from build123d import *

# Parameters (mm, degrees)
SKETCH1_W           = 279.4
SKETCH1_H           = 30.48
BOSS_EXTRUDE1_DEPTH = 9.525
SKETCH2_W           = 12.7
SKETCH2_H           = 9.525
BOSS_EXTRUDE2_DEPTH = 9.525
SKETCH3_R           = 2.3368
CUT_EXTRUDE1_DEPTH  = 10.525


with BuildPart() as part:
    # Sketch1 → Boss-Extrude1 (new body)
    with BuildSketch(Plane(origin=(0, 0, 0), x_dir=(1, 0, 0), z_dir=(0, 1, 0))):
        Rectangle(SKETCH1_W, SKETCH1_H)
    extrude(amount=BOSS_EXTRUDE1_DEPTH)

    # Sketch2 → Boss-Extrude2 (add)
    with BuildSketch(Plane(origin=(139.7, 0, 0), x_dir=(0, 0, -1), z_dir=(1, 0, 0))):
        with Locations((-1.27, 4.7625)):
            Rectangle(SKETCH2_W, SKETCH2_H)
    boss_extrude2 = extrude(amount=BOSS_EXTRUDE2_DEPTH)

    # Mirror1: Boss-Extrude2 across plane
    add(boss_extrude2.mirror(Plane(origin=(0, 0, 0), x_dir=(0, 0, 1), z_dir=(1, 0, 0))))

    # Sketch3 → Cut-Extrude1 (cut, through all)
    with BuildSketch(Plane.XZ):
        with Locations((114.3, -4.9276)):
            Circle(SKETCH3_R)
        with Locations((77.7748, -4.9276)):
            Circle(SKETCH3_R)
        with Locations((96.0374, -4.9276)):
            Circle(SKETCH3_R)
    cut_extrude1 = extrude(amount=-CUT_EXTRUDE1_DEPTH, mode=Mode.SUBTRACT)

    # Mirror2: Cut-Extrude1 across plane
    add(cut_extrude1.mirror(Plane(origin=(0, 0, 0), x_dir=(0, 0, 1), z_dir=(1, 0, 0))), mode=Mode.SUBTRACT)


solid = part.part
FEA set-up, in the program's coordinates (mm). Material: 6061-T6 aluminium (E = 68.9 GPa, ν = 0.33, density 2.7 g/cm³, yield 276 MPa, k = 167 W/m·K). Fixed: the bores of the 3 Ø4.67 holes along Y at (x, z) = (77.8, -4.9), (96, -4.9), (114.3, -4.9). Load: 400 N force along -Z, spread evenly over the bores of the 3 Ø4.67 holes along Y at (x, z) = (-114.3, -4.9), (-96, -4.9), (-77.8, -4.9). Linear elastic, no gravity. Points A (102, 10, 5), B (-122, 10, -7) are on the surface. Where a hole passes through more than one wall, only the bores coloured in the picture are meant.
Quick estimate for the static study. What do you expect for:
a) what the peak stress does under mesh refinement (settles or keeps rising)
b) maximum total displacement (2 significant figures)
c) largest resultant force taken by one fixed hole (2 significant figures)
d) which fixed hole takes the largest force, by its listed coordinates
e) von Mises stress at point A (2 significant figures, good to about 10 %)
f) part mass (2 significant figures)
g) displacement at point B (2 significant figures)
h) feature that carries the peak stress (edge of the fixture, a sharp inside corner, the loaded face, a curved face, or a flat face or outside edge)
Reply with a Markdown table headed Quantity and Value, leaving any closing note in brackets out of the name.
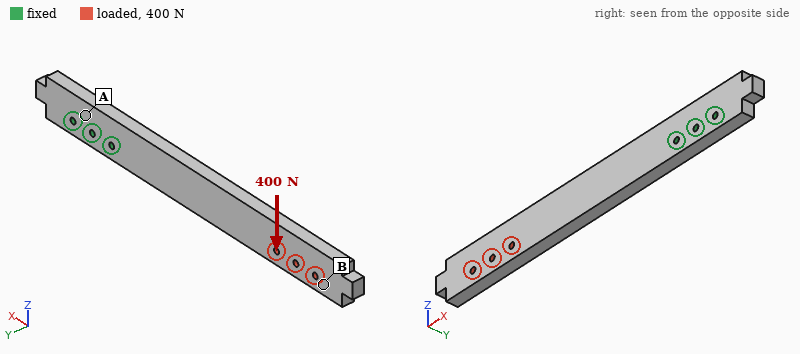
| Quantity | Value |
|---|---|
| what the peak stress does under mesh refinement | keeps rising |
| maximum total displacement | 0.81 mm |
| largest resultant force taken by one fixed hole | 2.8 kN |
| which fixed hole takes the largest force, by its listed coordinates | (77.8, -4.9) |
| von Mises stress at point A | 12 MPa |
| part mass | 220 g |
| displacement at point B | 0.69 mm |
| feature that carries the peak stress | edge of the fixture |
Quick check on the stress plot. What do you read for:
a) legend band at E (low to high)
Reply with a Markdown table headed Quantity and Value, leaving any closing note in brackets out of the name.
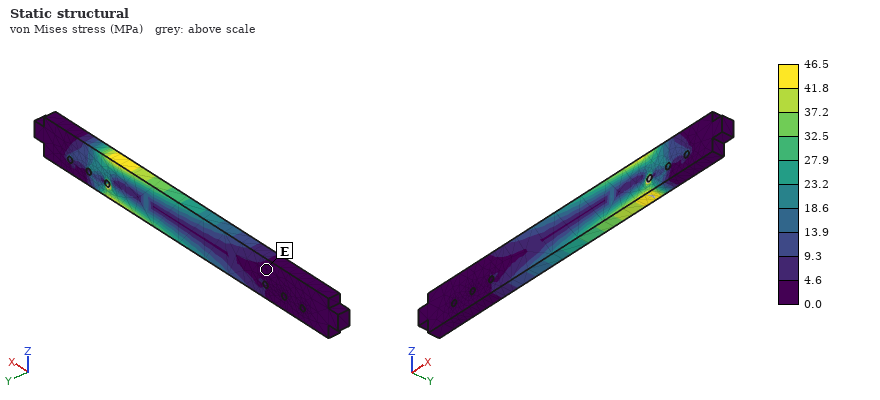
| Quantity | Value |
|---|---|
| legend band at E | 0.0 to 4.6 MPa |
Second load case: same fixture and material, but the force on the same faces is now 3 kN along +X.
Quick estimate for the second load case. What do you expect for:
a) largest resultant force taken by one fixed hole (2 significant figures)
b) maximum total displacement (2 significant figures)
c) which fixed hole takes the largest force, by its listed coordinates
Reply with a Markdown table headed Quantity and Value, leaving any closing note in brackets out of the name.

| Quantity | Value |
|---|---|
| largest resultant force taken by one fixed hole | 2.4 kN |
| maximum total displacement | 0.23 mm |
| which fixed hole takes the largest force, by its listed coordinates | (77.8, -4.9) |
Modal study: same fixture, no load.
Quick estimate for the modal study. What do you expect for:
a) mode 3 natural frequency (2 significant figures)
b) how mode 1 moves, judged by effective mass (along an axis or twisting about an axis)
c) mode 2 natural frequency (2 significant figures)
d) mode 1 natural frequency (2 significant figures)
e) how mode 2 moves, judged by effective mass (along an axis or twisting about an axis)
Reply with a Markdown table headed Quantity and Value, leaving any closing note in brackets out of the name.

| Quantity | Value |
|---|---|
| mode 3 natural frequency | 960 Hz |
| how mode 1 moves, judged by effective mass | along Y |
| mode 2 natural frequency | 450 Hz |
| mode 1 natural frequency | 160 Hz |
| how mode 2 moves, judged by effective mass | along Z |
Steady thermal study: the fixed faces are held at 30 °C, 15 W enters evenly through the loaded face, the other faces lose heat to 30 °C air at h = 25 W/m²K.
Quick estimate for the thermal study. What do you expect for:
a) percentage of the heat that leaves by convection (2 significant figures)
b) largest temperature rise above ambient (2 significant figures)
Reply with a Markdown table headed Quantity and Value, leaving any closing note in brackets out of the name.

| Quantity | Value |
|---|---|
| percentage of the heat that leaves by convection | 54 % |
| largest temperature rise above ambient | 31 K |
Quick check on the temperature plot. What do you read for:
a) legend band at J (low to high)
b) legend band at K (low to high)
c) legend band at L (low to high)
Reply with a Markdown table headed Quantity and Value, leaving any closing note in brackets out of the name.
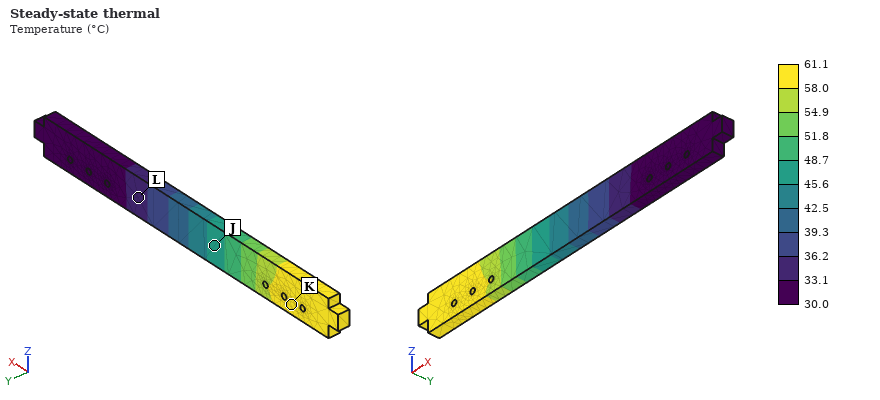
| Quantity | Value |
|---|---|
| legend band at J | 45.6 to 48.7 °C |
| legend band at K | 58.0 to 61.1 °C |
| legend band at L | 33.1 to 36.2 °C |
